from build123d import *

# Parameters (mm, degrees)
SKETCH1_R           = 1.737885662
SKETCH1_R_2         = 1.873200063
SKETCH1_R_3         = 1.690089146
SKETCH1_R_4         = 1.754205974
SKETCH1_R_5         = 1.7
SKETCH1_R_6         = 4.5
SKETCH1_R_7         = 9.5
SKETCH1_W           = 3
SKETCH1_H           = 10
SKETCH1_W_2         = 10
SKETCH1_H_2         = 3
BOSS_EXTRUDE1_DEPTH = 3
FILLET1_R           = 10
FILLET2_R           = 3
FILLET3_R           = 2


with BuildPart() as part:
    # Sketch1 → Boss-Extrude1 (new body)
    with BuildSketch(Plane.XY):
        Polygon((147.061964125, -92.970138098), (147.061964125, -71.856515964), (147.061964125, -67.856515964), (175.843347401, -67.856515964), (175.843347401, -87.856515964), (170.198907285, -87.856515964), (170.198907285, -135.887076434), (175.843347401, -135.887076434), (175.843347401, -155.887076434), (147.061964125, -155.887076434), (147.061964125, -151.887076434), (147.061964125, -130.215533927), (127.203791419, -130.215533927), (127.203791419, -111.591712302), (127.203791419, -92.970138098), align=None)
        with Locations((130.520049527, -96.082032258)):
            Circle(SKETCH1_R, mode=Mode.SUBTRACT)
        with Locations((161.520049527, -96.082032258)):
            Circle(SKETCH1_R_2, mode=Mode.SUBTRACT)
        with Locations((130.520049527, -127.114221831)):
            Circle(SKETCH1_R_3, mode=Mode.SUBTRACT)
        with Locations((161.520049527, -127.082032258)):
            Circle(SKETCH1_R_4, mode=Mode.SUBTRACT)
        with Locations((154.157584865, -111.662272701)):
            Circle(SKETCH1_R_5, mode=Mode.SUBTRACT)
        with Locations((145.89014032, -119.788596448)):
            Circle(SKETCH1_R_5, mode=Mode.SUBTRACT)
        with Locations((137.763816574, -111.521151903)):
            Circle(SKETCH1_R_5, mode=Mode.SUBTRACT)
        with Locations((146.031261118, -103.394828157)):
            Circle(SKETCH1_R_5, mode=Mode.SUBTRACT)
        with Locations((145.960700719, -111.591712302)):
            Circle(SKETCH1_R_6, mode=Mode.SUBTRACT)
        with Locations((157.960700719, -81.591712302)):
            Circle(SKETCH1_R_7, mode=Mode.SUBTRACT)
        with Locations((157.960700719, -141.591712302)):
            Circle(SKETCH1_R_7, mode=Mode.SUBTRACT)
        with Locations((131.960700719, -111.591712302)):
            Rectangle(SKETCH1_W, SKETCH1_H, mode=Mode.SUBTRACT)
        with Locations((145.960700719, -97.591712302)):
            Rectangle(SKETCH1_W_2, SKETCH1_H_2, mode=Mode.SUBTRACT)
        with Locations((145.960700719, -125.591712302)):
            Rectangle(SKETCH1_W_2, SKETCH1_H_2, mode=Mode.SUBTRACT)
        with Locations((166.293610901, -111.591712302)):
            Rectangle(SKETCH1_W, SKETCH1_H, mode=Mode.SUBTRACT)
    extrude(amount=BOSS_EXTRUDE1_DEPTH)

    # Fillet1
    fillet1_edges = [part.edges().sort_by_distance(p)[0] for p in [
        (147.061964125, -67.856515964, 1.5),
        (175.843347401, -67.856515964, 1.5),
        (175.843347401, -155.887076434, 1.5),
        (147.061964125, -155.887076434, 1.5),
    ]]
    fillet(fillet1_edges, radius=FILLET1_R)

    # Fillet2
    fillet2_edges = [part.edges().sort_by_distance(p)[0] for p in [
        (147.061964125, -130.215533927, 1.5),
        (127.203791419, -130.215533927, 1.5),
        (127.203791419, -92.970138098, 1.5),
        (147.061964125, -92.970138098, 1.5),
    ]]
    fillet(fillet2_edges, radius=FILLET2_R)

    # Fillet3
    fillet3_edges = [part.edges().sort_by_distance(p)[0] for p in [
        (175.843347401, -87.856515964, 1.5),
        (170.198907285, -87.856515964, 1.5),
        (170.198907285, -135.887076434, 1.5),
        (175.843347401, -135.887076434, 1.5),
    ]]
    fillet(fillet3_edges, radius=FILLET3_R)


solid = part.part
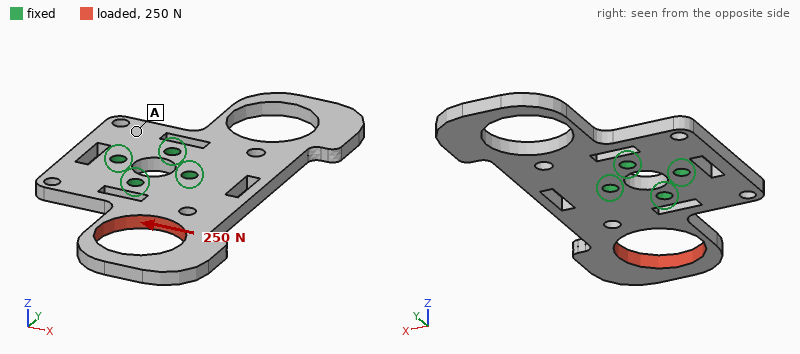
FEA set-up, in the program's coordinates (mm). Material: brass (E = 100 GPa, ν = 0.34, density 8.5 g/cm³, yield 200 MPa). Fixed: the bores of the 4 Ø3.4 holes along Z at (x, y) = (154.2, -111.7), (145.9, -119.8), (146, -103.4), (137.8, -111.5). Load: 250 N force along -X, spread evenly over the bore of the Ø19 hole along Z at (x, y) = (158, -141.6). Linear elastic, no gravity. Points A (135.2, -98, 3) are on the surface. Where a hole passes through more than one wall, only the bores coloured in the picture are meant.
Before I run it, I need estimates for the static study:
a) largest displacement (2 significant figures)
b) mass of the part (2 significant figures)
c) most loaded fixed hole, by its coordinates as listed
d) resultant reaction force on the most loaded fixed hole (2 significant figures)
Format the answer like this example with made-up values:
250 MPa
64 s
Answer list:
42 µm
53 g
(145.9, -119.8)
380 N
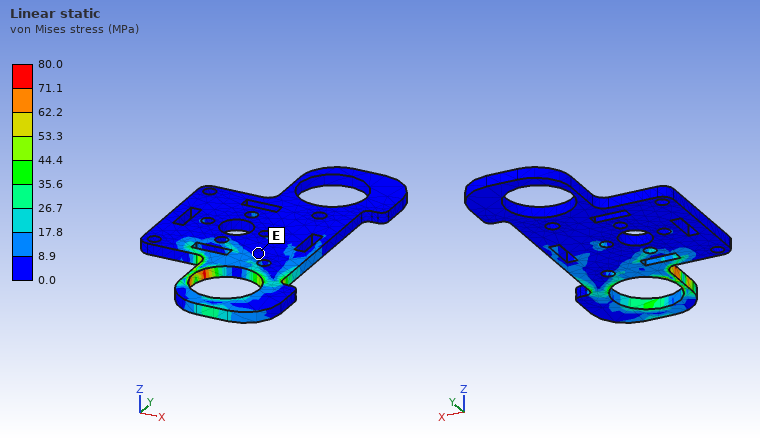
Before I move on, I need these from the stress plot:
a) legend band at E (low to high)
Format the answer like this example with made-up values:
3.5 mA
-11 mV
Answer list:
0.0 to 8.9 MPa
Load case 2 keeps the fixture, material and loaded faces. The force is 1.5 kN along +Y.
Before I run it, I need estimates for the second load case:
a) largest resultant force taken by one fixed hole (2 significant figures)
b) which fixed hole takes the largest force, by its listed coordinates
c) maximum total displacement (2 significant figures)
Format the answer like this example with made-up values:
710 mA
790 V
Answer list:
1.3 kN
(154.2, -111.7)
35 µm
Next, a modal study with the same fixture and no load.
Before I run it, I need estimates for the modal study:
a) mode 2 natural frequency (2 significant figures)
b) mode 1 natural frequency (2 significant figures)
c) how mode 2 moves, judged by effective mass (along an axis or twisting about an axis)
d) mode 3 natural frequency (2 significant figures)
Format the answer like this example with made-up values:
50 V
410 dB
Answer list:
1000 Hz
930 Hz
along Z
2700 Hz
